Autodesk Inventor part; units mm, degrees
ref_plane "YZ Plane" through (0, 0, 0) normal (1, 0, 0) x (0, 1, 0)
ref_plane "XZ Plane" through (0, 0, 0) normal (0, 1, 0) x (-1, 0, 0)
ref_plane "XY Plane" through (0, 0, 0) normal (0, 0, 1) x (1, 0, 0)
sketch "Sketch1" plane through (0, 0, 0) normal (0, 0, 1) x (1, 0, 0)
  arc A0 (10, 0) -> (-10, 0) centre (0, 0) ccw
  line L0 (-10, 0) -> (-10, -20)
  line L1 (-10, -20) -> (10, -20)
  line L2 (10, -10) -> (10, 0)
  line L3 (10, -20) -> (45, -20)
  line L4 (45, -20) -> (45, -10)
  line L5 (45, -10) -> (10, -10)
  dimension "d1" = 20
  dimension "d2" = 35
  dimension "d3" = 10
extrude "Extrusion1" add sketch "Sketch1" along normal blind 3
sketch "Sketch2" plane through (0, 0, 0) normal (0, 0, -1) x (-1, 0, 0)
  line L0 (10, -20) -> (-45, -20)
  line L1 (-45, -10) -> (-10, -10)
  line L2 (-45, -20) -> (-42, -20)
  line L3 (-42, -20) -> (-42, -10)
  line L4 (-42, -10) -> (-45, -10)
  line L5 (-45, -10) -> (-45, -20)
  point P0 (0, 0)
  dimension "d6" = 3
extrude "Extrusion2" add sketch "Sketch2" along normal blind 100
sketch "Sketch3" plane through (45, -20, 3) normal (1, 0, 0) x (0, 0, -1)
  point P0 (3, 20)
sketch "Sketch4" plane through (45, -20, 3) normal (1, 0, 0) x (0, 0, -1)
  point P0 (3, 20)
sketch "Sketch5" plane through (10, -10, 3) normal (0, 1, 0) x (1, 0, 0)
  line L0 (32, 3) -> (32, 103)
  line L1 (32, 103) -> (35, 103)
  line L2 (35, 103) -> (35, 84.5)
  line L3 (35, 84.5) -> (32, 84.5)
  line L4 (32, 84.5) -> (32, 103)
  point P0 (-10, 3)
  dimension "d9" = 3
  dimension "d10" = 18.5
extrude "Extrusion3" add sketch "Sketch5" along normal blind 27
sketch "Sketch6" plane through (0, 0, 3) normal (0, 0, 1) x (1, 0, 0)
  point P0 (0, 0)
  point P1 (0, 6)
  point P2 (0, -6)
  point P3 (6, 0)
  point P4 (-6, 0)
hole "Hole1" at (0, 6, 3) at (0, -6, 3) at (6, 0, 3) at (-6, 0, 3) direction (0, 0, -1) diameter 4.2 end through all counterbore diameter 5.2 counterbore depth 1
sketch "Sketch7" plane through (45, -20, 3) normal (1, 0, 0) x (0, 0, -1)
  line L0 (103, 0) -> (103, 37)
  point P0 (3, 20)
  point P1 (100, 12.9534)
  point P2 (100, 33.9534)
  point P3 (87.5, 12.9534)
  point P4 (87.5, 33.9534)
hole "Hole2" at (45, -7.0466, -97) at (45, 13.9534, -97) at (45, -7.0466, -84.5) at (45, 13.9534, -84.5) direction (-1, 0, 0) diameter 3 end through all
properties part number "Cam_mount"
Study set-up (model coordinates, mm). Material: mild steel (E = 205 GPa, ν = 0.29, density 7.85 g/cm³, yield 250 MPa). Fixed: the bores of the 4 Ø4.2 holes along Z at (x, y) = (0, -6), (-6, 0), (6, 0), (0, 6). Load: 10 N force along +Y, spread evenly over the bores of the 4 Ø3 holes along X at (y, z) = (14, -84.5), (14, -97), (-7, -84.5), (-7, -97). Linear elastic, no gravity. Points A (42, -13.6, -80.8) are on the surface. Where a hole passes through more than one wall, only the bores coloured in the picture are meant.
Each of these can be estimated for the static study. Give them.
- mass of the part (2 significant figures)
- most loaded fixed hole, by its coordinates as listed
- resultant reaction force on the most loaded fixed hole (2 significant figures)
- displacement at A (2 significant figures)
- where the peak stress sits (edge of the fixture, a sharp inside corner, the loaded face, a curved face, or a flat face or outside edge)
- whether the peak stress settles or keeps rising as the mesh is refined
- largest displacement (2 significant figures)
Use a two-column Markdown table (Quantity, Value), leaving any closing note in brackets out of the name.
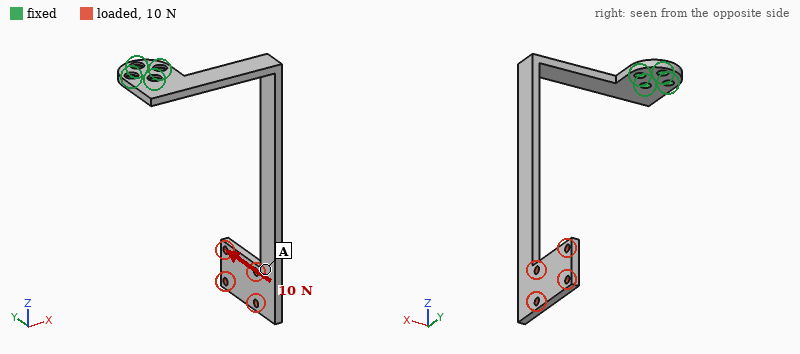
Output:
| Quantity | Value |
|---|---|
| mass of the part | 54 g |
| most loaded fixed hole, by its coordinates as listed | (0, -6) |
| resultant reaction force on the most loaded fixed hole | 110 N |
| displacement at A | 0.56 mm |
| where the peak stress sits | edge of the fixture |
| whether the peak stress settles or keeps rising as the mesh is refined | keeps rising |
| largest displacement | 0.72 mm |
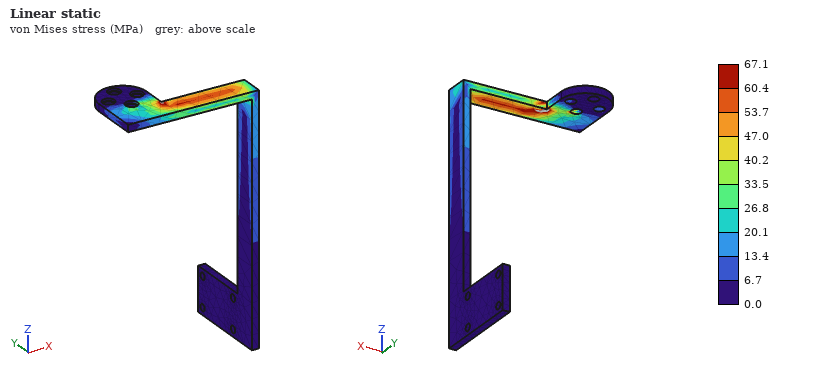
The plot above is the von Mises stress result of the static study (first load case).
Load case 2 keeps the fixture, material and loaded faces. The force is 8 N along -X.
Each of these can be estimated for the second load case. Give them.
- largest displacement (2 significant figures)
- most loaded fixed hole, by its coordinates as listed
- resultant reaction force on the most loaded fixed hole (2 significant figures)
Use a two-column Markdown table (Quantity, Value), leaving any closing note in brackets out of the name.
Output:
| Quantity | Value |
|---|---|
| largest displacement | 1.2 mm |
| most loaded fixed hole, by its coordinates as listed | (6, 0) |
| resultant reaction force on the most loaded fixed hole | 44 N |
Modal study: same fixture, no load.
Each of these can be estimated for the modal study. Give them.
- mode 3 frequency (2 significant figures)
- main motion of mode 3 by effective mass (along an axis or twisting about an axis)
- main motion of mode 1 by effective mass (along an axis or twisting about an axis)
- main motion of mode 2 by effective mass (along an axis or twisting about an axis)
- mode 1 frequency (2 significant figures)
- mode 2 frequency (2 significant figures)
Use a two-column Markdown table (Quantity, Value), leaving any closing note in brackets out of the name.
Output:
| Quantity | Value |
|---|---|
| mode 3 frequency | 470 Hz |
| main motion of mode 3 by effective mass | along Z |
| main motion of mode 1 by effective mass | along X |
| main motion of mode 2 by effective mass | along Y |
| mode 1 frequency | 97 Hz |
| mode 2 frequency | 140 Hz |
